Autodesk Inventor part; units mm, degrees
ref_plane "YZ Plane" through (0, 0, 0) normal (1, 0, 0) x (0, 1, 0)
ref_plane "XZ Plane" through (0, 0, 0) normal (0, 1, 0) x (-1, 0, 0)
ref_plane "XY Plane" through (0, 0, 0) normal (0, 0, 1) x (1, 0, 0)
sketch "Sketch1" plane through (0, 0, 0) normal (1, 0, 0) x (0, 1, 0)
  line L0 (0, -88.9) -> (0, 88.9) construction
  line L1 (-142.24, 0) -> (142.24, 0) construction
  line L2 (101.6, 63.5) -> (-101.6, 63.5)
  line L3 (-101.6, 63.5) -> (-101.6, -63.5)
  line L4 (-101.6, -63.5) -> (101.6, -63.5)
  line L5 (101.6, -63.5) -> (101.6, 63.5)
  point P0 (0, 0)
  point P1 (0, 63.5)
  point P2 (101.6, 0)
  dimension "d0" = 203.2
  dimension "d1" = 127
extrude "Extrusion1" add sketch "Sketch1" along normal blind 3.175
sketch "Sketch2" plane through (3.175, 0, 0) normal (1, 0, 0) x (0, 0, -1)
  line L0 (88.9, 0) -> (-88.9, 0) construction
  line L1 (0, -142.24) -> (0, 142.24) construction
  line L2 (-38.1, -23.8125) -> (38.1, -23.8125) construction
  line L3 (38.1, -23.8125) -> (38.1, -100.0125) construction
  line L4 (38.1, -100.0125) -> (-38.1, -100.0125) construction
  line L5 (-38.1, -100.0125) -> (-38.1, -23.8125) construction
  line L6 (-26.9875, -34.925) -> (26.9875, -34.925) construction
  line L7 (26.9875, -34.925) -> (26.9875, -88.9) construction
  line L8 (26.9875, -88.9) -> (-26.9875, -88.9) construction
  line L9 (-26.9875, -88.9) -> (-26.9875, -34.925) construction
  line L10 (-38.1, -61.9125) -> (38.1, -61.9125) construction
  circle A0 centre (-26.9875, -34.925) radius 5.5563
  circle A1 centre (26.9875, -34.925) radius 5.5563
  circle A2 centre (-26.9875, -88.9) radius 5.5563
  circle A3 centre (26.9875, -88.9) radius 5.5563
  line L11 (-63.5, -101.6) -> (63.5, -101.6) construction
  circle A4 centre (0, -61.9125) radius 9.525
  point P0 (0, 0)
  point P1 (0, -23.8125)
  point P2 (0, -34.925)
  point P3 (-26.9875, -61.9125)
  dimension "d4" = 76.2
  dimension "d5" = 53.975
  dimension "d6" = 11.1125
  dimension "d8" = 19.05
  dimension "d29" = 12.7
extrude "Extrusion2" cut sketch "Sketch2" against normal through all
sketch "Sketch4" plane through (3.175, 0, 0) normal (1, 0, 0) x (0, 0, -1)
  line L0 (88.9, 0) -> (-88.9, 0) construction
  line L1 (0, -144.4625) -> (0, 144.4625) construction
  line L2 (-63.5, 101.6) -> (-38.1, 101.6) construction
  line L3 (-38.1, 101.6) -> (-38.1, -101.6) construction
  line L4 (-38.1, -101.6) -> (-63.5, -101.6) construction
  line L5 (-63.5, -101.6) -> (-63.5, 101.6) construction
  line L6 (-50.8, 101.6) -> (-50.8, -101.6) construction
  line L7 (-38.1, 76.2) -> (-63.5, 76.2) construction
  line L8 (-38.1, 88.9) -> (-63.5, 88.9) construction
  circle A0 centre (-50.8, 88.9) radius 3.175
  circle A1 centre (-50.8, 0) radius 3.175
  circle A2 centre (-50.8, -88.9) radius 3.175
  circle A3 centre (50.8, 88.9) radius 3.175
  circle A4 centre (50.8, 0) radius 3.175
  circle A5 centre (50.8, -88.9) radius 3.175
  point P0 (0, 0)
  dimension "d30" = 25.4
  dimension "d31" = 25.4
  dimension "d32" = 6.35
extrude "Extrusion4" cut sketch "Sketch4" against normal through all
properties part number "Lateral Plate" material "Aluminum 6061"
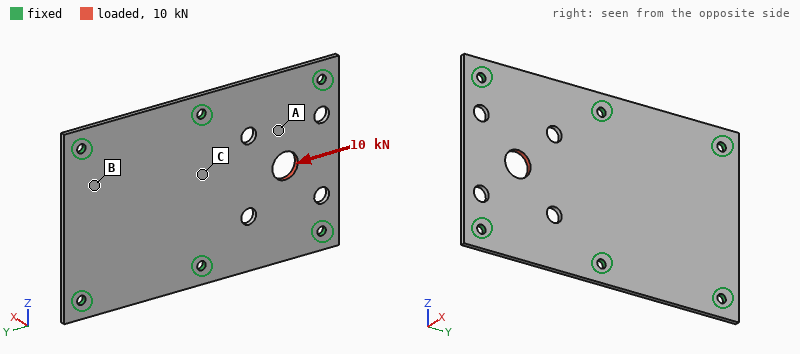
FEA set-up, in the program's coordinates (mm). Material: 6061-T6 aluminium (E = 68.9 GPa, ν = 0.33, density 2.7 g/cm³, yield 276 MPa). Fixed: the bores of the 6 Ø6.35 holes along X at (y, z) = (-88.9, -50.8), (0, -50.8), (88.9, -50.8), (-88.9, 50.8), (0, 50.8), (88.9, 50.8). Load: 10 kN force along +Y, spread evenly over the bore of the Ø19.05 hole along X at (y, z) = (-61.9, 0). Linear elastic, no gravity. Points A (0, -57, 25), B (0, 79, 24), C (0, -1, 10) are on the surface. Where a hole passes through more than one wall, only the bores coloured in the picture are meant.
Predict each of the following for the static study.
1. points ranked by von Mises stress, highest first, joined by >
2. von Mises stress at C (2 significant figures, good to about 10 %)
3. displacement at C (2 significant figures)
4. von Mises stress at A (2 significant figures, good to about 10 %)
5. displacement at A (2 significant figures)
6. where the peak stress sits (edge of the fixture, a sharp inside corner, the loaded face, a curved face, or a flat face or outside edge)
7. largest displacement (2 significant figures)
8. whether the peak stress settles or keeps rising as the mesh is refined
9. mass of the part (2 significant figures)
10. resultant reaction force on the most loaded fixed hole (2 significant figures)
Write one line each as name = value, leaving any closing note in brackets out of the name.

points ranked by von Mises stress, highest first, joined by > = A > C > B
von Mises stress at C = 16 MPa
displacement at C = 13 µm
von Mises stress at A = 34 MPa
displacement at A = 25 µm
where the peak stress sits = edge of the fixture
largest displacement = 52 µm
whether the peak stress settles or keeps rising as the mesh is refined = keeps rising
mass of the part = 210 g
resultant reaction force on the most loaded fixed hole = 2.4 kN
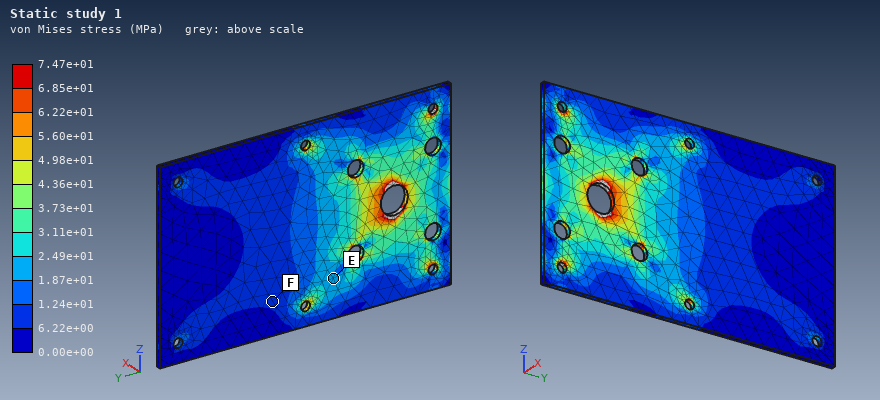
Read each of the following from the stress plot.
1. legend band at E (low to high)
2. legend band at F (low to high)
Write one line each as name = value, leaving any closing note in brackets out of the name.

legend band at E = 1.87e+01 to 2.49e+01 MPa
legend band at F = 6.22e+00 to 1.24e+01 MPa
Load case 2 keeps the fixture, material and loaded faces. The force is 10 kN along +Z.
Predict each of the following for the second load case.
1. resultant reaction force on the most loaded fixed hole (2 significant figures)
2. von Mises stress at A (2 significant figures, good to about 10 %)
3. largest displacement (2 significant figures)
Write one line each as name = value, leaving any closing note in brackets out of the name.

resultant reaction force on the most loaded fixed hole = 3.3 kN
von Mises stress at A = 28 MPa
largest displacement = 39 µm
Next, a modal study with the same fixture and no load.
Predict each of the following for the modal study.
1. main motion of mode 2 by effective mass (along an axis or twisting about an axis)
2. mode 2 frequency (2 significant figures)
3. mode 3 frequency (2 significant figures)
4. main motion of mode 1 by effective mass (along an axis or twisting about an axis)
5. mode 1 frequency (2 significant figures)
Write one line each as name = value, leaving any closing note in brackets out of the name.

main motion of mode 2 by effective mass = twisting about Z
mode 2 frequency = 1300 Hz
mode 3 frequency = 2000 Hz
main motion of mode 1 by effective mass = along X
mode 1 frequency = 1200 Hz
